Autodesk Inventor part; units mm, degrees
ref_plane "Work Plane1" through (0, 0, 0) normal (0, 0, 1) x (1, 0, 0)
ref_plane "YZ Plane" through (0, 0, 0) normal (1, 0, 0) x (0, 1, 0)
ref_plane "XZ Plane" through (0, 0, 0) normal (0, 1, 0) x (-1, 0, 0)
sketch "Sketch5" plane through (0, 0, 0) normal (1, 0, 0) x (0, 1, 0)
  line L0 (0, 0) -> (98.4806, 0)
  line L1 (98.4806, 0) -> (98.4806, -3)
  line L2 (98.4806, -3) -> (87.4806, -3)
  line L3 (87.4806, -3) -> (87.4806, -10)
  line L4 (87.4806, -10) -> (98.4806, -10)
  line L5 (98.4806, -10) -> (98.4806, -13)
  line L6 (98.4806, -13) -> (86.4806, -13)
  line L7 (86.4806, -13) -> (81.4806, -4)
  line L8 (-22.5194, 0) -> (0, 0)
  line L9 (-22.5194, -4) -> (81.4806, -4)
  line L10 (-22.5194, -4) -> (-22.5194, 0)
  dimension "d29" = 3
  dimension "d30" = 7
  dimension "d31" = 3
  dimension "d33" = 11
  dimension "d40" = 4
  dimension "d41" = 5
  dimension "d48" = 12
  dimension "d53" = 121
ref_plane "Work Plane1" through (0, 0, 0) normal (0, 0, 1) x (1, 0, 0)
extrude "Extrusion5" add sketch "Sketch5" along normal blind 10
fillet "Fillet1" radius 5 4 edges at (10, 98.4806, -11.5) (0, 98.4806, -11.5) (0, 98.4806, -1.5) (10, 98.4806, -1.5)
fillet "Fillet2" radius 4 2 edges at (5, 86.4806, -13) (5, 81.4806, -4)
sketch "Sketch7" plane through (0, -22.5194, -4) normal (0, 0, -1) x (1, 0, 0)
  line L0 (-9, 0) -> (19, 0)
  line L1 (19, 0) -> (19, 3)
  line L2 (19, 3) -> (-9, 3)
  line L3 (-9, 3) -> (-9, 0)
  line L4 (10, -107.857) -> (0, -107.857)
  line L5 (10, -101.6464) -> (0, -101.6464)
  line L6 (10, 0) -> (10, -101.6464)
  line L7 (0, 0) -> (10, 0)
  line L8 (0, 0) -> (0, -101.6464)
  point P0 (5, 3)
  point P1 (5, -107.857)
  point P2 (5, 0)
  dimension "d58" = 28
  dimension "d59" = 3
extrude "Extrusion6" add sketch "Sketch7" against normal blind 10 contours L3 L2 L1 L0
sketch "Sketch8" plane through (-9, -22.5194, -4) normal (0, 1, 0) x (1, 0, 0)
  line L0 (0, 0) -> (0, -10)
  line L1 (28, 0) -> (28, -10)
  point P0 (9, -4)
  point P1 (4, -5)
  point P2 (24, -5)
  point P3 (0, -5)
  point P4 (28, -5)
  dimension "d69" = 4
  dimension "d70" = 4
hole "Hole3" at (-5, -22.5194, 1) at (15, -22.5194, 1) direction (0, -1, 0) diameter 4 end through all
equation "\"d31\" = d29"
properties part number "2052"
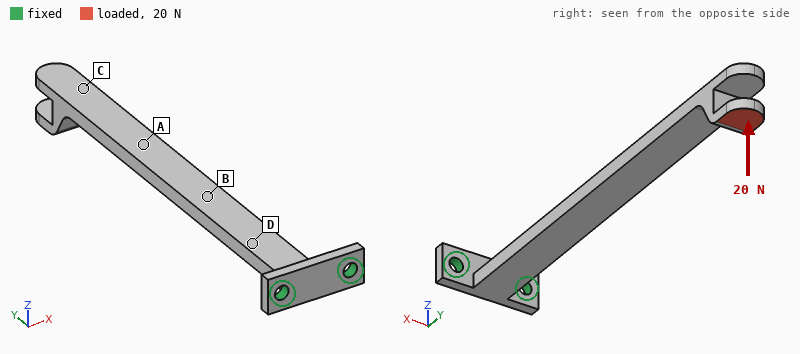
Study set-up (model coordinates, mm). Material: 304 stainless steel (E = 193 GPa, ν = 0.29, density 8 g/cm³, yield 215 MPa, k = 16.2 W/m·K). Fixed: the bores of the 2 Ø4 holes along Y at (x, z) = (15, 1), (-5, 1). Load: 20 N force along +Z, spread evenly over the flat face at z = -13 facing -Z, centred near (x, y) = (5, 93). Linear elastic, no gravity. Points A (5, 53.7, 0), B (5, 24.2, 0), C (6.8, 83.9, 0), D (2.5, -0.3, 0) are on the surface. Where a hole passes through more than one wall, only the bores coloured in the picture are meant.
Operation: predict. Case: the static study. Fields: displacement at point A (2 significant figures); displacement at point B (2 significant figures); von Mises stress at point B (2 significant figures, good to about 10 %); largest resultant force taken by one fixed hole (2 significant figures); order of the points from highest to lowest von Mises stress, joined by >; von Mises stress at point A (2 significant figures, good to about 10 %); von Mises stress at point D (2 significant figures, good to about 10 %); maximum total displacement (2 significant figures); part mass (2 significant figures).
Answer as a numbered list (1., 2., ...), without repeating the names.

1. 0.62 mm
2. 0.28 mm
3. 52 MPa
4. 28 N
5. D > B > A > C
6. 30 MPa
7. 70 MPa
8. 1.3 mm
9. 49 g
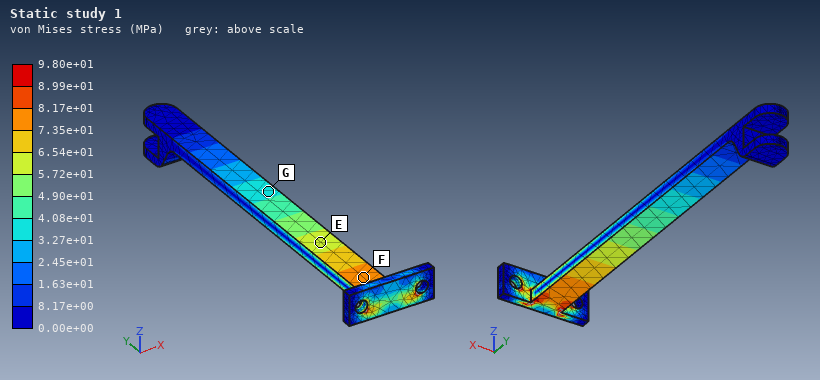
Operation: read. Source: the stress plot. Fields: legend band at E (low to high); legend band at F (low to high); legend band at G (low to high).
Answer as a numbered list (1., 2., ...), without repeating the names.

1. 5.72e+01 to 6.54e+01 MPa
2. 7.35e+01 to 8.17e+01 MPa
3. 3.27e+01 to 4.08e+01 MPa
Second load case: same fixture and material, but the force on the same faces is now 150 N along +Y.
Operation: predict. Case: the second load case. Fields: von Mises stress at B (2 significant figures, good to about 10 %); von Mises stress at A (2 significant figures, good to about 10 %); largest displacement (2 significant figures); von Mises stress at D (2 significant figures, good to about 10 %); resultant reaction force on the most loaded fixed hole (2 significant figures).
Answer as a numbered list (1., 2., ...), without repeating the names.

1. 58 MPa
2. 58 MPa
3. 1.3 mm
4. 58 MPa
5. 86 N
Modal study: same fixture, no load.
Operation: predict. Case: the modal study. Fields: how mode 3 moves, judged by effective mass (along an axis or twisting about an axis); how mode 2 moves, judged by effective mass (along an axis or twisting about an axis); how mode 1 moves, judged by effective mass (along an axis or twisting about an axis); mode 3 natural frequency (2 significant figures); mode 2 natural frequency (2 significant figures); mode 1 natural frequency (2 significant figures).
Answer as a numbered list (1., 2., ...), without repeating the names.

1. along Z
2. along X
3. along Z
4. 1200 Hz
5. 420 Hz
6. 170 Hz
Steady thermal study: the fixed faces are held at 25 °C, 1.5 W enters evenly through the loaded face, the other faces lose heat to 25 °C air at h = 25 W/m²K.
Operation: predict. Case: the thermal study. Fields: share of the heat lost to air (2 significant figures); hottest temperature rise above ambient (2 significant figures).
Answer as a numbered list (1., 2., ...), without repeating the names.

1. 98 %
2. 66 K
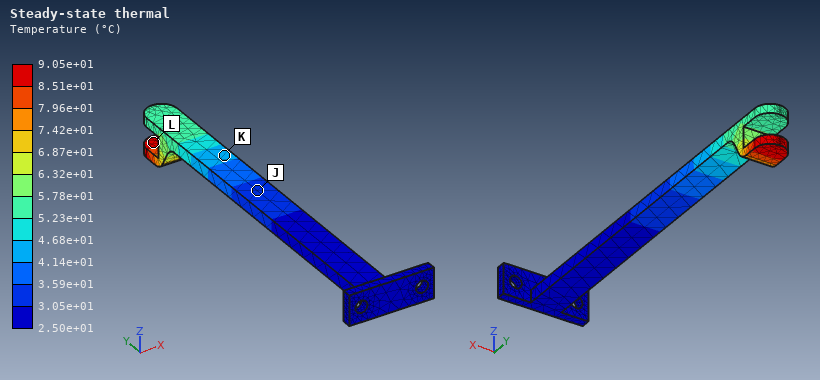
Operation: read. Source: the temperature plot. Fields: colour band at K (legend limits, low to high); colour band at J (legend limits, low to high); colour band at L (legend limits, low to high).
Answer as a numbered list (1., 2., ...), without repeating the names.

1. 4.14e+01 to 4.68e+01 °C
2. 3.05e+01 to 3.59e+01 °C
3. 8.51e+01 to 9.05e+01 °C
